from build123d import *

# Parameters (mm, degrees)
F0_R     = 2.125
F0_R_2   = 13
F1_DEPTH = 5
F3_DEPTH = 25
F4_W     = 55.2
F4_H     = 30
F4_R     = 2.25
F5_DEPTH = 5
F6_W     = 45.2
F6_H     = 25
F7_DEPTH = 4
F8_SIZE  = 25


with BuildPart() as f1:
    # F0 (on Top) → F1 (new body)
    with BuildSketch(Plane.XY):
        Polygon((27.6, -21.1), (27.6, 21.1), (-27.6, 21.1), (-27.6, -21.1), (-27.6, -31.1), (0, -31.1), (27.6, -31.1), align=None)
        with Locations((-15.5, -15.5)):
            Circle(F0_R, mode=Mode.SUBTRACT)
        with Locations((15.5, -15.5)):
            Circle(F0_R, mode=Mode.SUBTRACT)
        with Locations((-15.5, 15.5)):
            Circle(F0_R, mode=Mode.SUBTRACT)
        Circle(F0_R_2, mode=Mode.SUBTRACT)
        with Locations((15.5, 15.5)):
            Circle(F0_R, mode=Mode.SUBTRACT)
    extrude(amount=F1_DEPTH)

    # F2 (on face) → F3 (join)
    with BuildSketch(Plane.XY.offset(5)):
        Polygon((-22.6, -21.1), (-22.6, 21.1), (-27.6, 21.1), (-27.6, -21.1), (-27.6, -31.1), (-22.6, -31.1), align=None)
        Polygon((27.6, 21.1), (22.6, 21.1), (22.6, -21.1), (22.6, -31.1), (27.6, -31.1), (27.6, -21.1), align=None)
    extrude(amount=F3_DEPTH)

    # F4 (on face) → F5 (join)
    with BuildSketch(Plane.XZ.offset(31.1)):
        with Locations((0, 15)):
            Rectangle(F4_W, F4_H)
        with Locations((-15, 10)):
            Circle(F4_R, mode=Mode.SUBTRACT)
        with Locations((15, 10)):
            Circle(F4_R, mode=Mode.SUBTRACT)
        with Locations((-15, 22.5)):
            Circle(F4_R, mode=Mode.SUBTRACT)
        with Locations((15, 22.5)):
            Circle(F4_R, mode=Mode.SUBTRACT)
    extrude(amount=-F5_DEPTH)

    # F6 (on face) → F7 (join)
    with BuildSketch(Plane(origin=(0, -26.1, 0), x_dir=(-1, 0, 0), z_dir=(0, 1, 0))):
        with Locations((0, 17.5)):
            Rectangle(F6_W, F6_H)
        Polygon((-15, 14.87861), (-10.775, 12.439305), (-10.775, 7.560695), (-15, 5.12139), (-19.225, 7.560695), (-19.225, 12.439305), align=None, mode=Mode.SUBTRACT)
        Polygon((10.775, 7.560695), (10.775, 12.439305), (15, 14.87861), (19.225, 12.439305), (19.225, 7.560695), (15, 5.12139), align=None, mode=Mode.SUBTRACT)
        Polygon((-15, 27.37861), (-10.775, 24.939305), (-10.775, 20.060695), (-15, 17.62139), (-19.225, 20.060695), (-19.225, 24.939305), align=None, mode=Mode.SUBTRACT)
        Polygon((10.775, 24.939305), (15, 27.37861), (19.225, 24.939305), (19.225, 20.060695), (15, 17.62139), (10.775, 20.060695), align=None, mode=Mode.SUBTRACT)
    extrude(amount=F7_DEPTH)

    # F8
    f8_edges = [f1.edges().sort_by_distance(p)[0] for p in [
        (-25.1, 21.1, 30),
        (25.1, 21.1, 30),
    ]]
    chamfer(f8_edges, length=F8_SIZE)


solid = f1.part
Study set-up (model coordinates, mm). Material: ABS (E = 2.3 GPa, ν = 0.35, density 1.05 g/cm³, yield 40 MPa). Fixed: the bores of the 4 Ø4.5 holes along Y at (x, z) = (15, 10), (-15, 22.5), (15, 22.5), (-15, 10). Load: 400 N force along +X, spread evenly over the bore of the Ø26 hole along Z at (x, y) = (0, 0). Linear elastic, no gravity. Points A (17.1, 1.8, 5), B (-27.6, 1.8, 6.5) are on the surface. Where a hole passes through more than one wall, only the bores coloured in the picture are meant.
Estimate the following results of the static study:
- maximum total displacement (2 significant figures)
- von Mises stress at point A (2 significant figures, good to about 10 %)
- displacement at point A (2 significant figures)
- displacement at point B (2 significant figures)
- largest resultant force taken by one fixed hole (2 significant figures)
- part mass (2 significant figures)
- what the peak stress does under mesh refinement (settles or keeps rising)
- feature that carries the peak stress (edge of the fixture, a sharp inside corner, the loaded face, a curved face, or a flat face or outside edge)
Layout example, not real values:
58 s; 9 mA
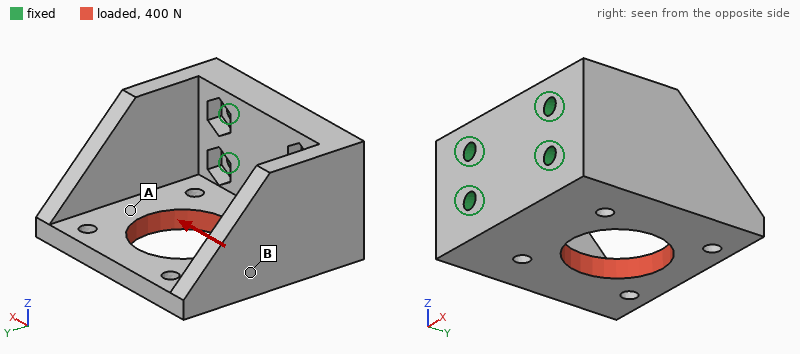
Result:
0.40 mm; 4.1 MPa; 0.23 mm; 0.26 mm; 360 N; 32 g; keeps rising; edge of the fixture
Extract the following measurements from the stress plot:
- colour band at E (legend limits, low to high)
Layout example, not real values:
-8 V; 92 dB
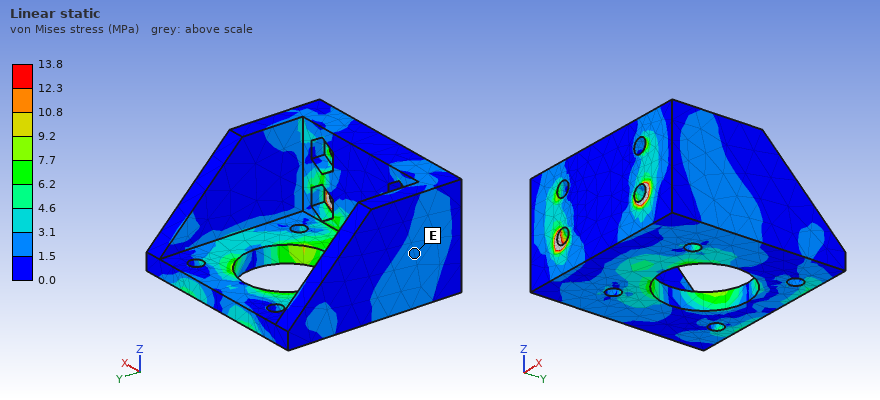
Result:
1.5 to 3.1 MPa
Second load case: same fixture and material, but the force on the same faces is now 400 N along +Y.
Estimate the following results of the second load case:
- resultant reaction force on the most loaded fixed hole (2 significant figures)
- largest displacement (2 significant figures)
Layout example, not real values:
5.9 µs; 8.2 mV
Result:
260 N; 0.18 mm
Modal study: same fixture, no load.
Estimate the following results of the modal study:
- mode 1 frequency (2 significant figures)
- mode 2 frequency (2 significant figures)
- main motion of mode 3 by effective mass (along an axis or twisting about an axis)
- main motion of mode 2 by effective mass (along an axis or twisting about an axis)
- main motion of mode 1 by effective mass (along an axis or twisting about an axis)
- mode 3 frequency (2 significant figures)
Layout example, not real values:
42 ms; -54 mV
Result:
1300 Hz; 1400 Hz; along X; along X; along Z; 2100 Hz
